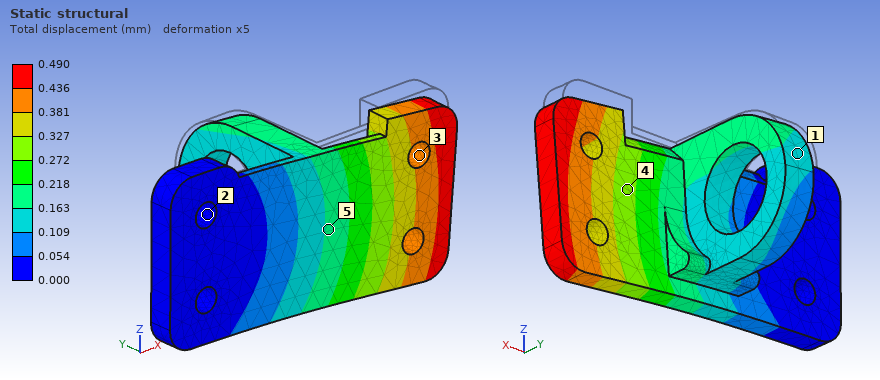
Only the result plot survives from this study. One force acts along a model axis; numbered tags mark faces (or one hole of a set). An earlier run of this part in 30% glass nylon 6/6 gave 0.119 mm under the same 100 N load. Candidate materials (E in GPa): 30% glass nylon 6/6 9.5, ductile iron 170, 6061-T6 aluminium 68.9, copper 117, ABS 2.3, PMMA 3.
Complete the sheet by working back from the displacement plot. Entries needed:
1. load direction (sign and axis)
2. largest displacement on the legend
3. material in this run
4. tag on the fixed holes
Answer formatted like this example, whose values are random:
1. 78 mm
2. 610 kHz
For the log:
1. -Z
2. 0.490 mm
3. ABS
4. 2
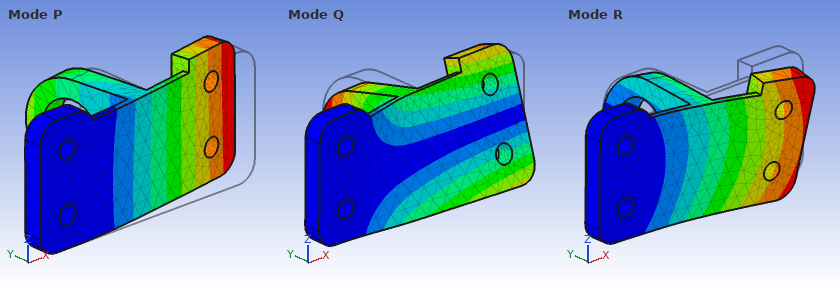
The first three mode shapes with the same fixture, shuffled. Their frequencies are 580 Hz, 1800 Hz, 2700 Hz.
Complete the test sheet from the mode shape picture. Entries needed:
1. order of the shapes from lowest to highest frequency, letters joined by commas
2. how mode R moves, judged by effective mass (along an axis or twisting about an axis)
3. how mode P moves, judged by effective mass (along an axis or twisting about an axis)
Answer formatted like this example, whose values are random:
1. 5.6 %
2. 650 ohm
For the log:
1. P, Q, R
2. along Z
3. along Y
